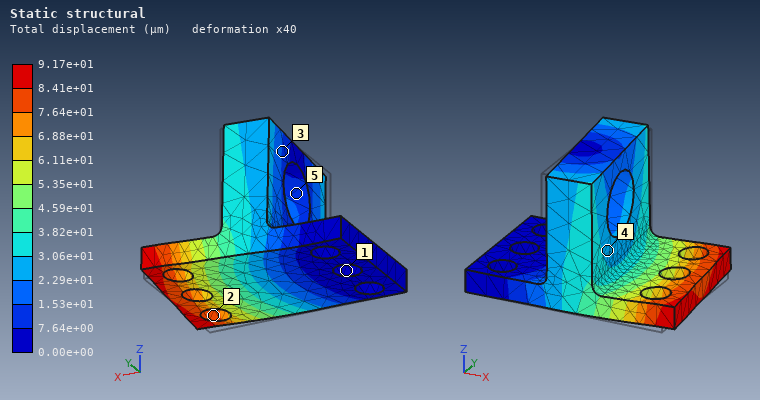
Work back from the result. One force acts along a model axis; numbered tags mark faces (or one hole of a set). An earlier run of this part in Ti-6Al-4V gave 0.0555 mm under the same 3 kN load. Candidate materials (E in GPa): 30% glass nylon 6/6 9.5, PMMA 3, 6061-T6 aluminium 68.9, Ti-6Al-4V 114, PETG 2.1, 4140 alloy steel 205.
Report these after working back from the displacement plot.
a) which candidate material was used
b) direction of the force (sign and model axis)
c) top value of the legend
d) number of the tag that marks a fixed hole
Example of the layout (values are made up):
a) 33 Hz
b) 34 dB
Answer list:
a) 6061-T6 aluminium
b) +Y
c) 9.17e+01 µm
d) 1
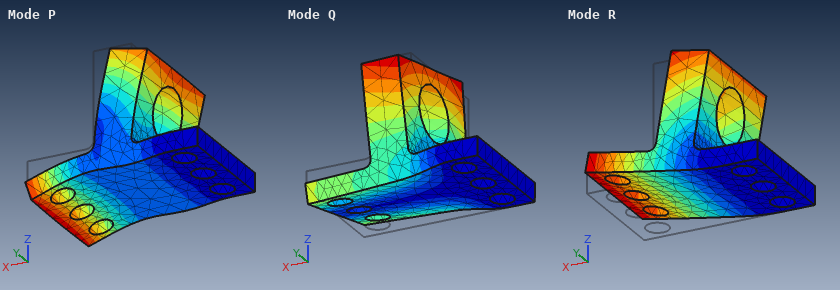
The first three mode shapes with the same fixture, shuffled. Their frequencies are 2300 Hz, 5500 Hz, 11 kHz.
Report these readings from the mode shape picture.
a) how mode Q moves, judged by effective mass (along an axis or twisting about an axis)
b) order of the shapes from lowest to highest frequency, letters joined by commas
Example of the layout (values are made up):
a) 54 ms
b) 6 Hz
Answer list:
a) along Y
b) R, Q, P
